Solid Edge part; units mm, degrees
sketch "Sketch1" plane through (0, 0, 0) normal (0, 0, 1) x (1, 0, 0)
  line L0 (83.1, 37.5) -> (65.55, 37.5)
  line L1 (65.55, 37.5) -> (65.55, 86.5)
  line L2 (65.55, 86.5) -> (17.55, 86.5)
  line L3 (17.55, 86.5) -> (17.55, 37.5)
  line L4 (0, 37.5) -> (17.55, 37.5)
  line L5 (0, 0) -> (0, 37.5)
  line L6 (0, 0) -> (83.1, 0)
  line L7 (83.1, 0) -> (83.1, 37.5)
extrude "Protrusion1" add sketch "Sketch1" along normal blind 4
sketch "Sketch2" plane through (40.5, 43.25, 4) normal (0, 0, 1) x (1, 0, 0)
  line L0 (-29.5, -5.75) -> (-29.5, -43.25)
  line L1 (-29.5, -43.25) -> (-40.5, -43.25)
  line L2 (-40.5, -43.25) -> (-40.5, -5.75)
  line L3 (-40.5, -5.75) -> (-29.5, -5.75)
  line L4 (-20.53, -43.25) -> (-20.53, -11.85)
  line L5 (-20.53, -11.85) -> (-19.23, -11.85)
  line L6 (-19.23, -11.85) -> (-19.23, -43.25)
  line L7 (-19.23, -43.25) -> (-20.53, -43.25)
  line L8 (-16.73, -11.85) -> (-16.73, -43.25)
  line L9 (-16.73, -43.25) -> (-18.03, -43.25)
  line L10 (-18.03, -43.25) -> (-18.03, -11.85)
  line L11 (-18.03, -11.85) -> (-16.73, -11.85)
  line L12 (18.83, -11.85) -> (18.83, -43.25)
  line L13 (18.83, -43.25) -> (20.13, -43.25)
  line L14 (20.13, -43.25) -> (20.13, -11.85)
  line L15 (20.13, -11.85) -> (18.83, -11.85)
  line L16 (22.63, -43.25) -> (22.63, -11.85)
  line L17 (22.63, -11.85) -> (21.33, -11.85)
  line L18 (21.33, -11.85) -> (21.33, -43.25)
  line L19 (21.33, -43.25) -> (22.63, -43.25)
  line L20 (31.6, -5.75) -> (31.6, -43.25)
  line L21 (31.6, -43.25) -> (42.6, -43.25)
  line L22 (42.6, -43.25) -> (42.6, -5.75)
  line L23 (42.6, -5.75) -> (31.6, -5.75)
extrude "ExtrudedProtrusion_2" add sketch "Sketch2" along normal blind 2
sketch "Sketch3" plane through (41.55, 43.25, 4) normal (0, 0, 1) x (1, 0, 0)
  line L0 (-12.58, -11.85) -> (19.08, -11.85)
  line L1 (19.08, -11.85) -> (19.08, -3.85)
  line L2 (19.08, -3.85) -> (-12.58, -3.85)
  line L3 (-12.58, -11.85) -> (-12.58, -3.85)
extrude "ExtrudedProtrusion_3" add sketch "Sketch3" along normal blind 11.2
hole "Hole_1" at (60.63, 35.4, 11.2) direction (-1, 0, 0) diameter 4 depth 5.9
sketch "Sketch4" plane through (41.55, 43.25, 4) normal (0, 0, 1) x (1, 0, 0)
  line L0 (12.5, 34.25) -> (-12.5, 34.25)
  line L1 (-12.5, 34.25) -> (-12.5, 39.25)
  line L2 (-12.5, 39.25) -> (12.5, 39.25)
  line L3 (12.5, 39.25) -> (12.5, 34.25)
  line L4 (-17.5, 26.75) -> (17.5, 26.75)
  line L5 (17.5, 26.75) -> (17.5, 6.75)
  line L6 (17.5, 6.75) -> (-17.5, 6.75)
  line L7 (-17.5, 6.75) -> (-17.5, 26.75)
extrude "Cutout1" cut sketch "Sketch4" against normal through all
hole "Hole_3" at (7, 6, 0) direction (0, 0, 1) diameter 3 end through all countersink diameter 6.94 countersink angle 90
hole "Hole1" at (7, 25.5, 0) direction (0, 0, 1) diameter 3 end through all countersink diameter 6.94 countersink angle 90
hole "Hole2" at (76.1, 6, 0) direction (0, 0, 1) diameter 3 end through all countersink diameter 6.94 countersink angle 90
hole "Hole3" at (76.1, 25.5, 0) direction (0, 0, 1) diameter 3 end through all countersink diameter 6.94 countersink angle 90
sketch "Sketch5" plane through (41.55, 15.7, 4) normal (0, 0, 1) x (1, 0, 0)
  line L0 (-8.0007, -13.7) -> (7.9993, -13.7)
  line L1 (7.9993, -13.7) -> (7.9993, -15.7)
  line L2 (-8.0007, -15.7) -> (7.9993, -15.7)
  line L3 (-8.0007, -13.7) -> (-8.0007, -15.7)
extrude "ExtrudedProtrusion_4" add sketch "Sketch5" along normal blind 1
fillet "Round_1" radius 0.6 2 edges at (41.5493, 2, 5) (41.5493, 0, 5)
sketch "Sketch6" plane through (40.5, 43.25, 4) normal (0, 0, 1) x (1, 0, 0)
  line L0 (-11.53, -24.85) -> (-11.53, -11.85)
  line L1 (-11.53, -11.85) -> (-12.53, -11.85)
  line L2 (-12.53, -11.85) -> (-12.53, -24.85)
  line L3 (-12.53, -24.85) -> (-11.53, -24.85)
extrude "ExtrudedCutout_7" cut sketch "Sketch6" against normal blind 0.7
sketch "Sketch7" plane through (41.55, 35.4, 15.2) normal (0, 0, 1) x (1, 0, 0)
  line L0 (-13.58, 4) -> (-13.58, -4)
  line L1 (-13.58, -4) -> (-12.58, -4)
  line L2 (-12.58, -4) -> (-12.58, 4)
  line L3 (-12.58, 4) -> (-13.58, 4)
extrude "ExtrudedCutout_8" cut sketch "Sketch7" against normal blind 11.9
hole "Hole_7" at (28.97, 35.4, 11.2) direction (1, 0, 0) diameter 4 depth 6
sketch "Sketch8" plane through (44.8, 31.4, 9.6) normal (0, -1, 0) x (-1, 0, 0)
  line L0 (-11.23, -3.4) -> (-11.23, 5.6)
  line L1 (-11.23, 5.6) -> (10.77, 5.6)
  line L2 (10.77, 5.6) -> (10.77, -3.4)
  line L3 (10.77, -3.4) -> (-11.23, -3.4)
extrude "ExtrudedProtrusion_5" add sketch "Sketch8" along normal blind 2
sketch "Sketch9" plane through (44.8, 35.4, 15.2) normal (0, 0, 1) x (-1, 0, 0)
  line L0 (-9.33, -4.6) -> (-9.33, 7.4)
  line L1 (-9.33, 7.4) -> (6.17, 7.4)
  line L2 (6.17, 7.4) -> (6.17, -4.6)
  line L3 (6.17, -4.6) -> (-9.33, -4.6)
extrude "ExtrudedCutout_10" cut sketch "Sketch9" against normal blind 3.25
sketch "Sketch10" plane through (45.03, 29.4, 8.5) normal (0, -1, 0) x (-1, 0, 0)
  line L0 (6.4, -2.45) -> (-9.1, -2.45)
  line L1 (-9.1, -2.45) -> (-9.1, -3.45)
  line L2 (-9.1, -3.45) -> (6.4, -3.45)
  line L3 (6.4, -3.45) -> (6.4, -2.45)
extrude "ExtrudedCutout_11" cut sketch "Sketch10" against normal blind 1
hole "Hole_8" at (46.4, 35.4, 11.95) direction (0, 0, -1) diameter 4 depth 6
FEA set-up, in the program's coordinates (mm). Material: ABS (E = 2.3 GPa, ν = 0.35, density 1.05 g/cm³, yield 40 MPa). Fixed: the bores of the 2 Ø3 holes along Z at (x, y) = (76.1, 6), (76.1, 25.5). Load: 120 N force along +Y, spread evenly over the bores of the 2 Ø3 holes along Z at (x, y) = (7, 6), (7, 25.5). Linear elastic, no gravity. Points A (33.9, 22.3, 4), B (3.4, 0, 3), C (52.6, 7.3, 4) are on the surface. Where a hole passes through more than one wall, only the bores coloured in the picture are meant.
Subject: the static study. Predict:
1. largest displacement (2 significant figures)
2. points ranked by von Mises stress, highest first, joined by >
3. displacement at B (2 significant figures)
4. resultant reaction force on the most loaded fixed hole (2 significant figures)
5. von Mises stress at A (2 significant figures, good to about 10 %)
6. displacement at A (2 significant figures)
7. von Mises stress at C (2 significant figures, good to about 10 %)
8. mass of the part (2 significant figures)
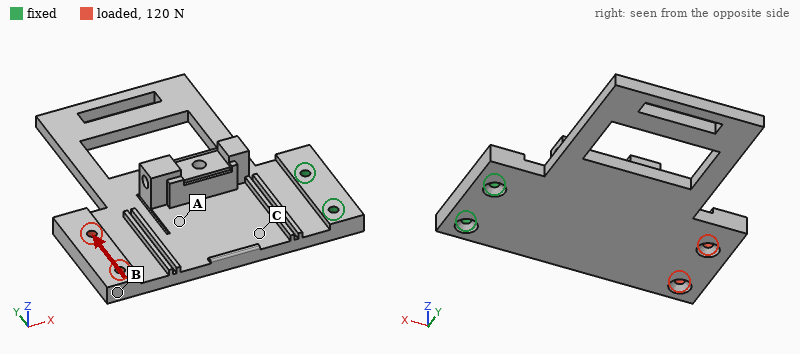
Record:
1.1 mm
C > A > B
0.62 mm
400 N
3.1 MPa
0.33 mm
5.0 MPa
24 g
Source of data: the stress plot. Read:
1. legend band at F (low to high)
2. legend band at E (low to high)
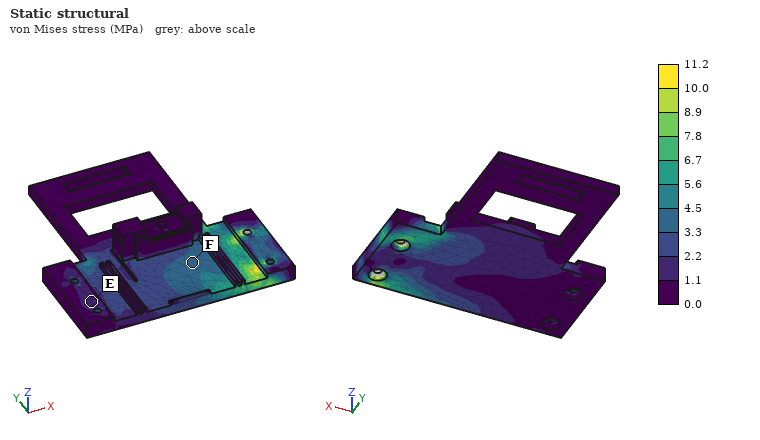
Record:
3.3 to 4.5 MPa
1.1 to 2.2 MPa
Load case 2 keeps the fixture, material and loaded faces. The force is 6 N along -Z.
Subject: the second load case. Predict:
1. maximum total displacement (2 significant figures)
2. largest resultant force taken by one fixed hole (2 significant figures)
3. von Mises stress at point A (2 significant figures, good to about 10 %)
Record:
1.2 mm
5.1 N
0.99 MPa
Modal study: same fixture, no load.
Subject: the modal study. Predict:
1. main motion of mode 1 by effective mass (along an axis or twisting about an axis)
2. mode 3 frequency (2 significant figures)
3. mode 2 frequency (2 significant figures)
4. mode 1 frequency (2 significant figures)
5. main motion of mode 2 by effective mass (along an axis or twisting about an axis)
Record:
along Z
610 Hz
230 Hz
140 Hz
twisting about X
